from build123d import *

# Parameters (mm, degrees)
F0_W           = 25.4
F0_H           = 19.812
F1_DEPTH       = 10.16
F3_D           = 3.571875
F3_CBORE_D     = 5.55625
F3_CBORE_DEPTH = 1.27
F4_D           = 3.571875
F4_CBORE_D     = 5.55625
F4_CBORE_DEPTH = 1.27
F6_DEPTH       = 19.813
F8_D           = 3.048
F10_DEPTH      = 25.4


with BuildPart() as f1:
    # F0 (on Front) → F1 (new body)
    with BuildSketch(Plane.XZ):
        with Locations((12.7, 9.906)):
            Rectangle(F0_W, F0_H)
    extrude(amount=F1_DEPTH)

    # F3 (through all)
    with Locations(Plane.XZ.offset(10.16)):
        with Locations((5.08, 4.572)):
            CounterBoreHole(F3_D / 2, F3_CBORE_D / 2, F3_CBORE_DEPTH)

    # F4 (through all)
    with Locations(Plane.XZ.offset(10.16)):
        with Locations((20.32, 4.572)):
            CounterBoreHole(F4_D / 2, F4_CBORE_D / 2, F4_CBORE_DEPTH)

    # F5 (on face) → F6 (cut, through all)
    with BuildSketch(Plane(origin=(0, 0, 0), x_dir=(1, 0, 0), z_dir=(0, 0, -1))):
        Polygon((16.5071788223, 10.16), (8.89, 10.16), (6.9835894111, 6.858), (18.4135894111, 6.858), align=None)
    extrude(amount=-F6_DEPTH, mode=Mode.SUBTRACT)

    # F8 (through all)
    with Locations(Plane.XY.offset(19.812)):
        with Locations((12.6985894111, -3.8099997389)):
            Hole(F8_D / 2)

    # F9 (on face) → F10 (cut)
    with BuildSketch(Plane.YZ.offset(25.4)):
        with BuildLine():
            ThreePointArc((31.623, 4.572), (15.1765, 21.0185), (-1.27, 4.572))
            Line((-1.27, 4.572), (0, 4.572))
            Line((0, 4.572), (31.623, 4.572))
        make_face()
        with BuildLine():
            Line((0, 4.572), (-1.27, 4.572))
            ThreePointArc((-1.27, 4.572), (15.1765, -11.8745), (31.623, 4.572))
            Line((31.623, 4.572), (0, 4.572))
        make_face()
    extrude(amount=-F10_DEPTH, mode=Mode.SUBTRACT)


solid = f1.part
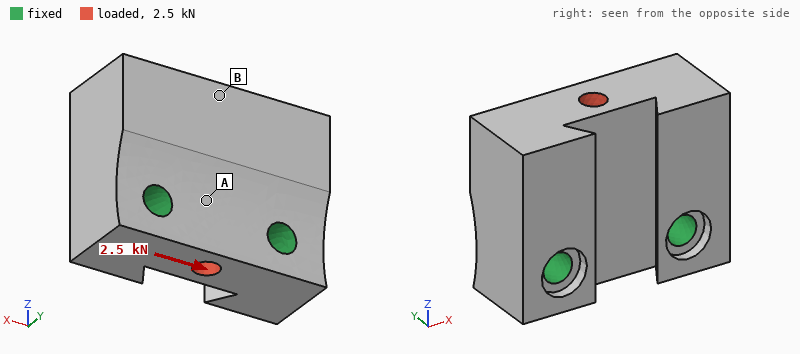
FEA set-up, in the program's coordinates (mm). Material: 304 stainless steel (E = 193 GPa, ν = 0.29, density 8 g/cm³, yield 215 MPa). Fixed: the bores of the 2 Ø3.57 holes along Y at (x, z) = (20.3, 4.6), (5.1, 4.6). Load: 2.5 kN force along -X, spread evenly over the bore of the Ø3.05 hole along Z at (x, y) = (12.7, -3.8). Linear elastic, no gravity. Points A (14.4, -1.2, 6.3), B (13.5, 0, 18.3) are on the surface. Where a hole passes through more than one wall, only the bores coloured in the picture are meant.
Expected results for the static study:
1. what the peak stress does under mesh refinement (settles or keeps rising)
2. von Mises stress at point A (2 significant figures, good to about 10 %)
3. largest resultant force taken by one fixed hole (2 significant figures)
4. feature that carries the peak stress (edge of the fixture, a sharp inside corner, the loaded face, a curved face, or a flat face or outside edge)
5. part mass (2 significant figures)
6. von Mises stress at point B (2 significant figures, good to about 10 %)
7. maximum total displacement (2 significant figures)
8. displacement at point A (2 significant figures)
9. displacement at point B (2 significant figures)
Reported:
keeps rising
18 MPa
1.4 kN
edge of the fixture
31 g
6.5 MPa
2.3 µm
0.61 µm
1.8 µm
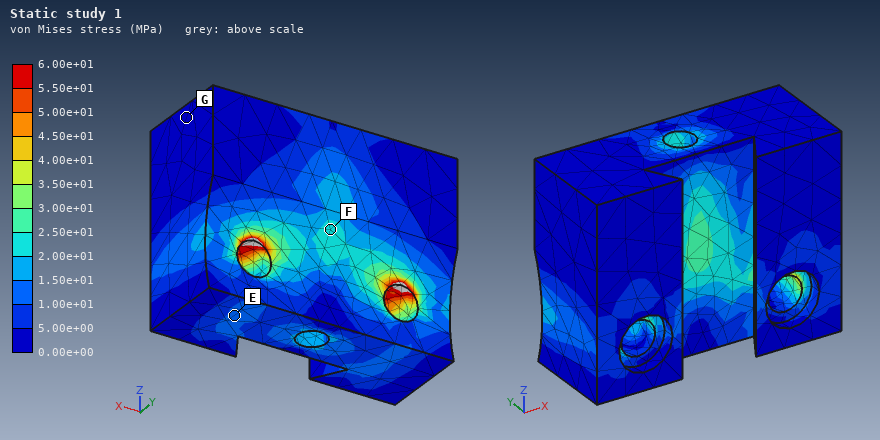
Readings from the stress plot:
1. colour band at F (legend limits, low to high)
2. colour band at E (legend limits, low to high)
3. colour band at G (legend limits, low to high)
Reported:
2.00e+01 to 2.50e+01 MPa
1.00e+01 to 1.50e+01 MPa
0.00e+00 to 5.00e+00 MPa
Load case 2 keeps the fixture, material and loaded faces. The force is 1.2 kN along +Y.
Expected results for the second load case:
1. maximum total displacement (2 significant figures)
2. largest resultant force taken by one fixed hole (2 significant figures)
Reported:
3.8 µm
600 N
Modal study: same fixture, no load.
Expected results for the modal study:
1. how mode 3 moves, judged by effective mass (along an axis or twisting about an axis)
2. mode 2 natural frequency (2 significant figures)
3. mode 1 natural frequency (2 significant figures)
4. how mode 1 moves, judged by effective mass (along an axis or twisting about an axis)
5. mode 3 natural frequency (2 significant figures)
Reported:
along X
28 kHz
21 kHz
along Y
34 kHz
